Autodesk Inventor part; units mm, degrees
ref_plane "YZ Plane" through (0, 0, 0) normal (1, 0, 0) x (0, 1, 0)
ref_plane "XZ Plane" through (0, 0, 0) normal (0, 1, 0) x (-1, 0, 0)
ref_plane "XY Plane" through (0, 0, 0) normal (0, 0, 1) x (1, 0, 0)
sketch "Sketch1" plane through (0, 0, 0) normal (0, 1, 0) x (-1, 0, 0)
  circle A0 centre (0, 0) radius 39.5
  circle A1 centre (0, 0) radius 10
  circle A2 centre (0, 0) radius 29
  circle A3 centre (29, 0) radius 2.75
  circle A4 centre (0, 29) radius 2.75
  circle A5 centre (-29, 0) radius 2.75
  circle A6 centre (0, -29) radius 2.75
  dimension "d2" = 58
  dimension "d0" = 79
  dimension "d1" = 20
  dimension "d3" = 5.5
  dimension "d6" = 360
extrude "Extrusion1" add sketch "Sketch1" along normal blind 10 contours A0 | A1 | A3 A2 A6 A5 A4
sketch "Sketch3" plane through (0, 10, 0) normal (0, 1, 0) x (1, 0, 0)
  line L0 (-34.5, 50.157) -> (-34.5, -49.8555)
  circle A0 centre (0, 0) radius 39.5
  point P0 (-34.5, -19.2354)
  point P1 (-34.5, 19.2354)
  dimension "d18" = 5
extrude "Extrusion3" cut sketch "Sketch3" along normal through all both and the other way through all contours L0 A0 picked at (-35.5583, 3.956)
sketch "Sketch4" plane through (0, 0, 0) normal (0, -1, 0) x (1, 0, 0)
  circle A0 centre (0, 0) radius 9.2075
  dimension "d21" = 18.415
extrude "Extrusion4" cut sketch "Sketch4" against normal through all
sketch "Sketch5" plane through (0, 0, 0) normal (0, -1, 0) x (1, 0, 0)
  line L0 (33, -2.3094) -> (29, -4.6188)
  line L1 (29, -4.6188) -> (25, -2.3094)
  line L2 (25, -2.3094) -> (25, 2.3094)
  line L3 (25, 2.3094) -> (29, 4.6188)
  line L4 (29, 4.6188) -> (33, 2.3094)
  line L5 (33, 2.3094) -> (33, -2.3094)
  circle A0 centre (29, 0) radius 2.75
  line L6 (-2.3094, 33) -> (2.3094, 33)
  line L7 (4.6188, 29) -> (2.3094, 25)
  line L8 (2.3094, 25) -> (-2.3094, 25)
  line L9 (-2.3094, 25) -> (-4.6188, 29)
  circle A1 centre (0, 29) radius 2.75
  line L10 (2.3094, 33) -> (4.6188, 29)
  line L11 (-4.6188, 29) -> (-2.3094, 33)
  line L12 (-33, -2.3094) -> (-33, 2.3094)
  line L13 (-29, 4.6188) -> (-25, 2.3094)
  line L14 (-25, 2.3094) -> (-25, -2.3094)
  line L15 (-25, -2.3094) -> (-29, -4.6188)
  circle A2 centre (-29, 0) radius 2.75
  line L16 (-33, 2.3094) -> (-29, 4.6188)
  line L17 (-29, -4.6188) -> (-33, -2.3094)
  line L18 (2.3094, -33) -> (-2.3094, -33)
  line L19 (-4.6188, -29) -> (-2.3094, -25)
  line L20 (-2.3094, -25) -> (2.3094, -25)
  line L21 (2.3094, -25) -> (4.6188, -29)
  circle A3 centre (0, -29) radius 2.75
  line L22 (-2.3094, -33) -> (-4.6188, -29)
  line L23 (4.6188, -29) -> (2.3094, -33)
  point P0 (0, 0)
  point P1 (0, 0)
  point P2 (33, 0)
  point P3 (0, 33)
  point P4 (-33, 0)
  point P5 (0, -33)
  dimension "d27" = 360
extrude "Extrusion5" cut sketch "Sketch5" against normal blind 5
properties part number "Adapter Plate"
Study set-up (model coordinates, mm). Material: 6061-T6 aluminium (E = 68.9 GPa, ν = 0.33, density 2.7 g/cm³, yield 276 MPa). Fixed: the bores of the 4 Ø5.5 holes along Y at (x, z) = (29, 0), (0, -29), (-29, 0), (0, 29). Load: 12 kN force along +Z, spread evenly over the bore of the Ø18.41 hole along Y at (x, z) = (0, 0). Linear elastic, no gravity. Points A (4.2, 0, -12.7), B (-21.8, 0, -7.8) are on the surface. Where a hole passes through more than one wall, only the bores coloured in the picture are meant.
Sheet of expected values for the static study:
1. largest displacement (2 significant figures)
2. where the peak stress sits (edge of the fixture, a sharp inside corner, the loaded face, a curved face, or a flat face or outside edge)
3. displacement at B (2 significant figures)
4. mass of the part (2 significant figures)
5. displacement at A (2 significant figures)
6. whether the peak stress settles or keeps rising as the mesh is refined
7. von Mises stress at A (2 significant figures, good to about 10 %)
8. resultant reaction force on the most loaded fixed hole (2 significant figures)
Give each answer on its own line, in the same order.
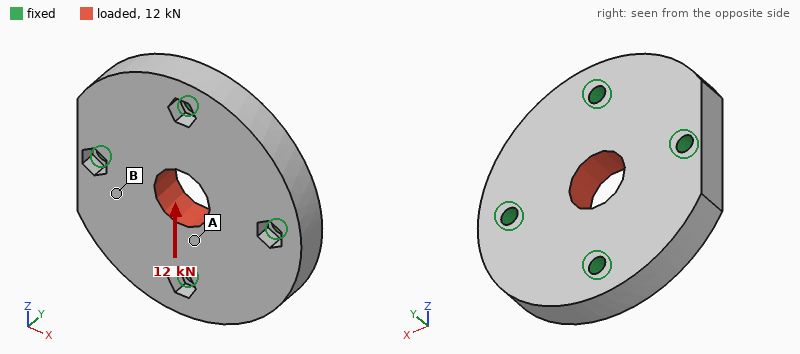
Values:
9.5 µm
edge of the fixture
4.7 µm
120 g
7.8 µm
keeps rising
25 MPa
3.7 kN
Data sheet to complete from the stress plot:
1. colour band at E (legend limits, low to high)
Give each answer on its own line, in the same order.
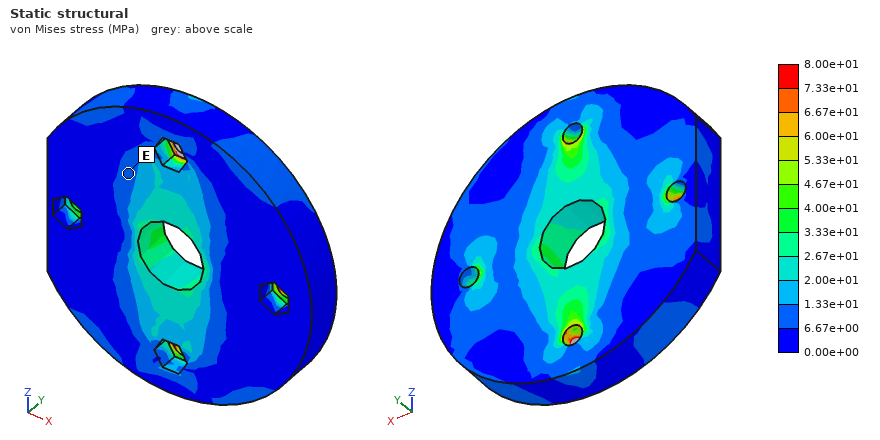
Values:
6.67e+00 to 1.33e+01 MPa
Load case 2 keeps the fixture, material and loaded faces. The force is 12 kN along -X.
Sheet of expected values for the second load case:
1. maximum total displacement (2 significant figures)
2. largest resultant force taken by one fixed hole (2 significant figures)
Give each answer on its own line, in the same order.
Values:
9.6 µm
3.7 kN
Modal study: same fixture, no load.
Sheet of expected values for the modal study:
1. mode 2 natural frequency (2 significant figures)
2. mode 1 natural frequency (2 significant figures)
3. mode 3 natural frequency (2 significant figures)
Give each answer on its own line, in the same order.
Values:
13 kHz
11 kHz
13 kHz
